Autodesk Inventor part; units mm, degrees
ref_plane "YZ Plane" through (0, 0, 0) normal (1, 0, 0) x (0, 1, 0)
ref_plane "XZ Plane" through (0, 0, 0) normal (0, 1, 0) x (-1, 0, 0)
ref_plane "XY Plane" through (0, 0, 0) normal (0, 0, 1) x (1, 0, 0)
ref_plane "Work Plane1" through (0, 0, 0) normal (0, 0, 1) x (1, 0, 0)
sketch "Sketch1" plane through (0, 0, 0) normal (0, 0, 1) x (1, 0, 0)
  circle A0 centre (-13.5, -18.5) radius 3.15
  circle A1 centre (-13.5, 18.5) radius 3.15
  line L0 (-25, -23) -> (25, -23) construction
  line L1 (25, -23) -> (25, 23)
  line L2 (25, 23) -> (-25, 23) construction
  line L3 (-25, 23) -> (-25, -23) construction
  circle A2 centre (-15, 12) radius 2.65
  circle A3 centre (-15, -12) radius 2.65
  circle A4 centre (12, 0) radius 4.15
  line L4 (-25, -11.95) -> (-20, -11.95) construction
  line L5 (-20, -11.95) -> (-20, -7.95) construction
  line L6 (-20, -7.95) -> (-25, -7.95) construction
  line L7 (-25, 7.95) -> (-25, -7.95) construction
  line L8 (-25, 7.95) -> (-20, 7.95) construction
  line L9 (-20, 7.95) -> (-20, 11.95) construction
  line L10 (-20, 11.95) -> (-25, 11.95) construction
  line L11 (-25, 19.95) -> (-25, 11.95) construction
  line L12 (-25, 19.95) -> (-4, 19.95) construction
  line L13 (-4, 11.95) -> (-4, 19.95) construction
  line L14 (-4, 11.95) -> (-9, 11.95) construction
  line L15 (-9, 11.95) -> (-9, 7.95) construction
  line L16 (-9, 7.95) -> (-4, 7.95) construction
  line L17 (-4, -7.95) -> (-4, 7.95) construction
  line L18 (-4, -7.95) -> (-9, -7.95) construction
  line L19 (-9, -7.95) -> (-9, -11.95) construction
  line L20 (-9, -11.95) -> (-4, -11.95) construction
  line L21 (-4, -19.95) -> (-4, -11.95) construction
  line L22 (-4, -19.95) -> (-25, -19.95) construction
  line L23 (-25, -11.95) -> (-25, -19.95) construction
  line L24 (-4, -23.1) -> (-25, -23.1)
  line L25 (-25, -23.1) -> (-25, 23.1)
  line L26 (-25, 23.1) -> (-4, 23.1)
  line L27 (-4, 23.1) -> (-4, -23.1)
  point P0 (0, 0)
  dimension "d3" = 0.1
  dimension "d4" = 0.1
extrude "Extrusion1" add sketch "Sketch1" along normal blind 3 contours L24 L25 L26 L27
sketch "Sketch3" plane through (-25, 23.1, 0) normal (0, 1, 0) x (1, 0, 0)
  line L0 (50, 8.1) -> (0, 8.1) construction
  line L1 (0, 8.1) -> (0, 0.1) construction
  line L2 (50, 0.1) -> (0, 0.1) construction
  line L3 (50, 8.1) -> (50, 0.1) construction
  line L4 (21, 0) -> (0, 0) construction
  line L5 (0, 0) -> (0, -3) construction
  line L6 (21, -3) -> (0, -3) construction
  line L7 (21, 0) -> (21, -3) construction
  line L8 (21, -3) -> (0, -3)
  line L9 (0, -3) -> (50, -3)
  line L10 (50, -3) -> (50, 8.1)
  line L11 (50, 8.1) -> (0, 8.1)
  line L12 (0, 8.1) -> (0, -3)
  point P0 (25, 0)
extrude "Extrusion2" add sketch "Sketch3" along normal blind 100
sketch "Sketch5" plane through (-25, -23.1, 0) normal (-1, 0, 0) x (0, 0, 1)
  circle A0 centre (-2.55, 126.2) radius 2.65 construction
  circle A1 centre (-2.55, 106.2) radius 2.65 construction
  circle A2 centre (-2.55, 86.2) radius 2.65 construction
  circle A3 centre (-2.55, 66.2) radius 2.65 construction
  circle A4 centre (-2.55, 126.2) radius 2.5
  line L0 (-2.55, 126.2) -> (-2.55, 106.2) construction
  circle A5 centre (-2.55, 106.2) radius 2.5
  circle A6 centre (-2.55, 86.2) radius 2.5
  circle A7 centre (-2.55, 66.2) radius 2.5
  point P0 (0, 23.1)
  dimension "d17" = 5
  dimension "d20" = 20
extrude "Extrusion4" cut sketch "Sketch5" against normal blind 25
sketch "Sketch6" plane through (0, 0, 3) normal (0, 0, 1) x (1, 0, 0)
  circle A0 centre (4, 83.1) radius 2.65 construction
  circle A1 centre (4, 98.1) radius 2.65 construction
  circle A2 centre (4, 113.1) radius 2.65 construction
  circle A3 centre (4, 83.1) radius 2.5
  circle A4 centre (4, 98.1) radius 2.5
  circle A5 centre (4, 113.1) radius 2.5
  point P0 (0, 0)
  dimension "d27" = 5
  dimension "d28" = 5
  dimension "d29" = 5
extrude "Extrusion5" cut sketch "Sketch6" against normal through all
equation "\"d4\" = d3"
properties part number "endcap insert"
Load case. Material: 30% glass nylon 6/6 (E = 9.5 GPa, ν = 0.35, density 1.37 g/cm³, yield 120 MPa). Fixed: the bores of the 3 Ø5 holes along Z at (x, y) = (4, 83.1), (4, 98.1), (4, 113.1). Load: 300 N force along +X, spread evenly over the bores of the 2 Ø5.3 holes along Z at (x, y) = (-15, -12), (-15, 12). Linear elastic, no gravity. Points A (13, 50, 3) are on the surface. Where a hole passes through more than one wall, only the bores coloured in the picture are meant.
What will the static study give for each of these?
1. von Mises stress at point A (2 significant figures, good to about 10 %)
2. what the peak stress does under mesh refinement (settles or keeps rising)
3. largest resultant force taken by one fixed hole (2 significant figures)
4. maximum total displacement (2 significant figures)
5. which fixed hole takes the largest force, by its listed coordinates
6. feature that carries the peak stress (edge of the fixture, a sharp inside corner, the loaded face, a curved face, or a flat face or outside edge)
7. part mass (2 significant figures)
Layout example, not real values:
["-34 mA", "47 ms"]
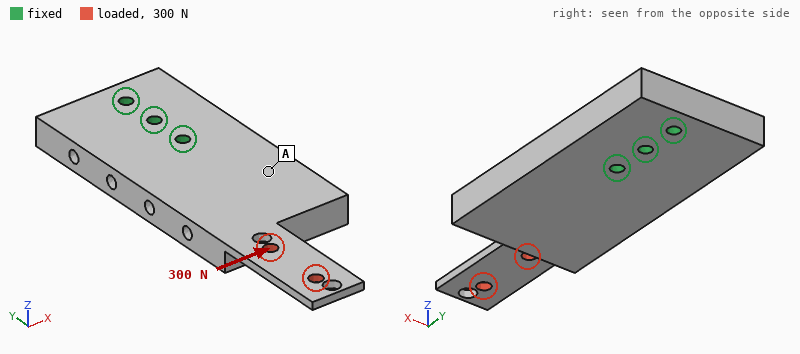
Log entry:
["3.2 MPa", "keeps rising", "1.1 kN", "0.55 mm", "(4, 83.1)", "a sharp inside corner", "76 g"]
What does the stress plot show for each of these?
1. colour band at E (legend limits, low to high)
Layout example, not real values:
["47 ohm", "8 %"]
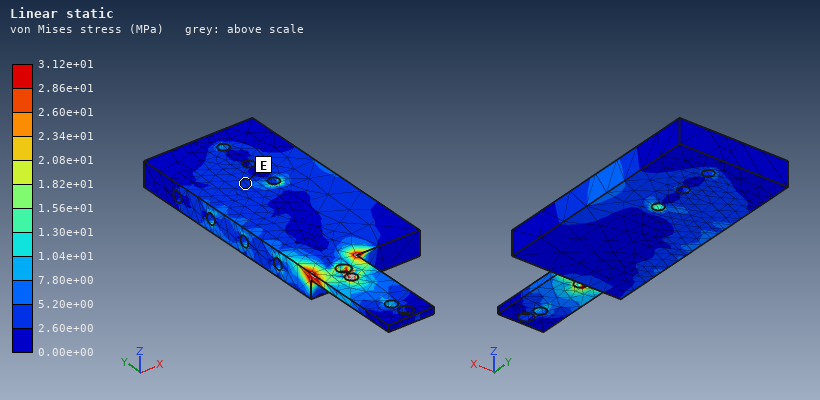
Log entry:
["2.60e+00 to 5.20e+00 MPa"]
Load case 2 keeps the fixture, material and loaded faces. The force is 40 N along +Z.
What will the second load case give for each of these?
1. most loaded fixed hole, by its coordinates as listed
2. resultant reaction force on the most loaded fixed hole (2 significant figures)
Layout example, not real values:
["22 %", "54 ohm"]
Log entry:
["(4, 83.1)", "120 N"]
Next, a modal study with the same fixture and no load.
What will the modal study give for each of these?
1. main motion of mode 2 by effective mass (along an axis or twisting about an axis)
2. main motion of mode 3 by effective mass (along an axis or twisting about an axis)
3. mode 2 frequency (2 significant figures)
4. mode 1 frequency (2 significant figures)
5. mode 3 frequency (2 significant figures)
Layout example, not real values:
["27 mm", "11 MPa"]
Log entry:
["along Z", "along X", "1200 Hz", "500 Hz", "1900 Hz"]
